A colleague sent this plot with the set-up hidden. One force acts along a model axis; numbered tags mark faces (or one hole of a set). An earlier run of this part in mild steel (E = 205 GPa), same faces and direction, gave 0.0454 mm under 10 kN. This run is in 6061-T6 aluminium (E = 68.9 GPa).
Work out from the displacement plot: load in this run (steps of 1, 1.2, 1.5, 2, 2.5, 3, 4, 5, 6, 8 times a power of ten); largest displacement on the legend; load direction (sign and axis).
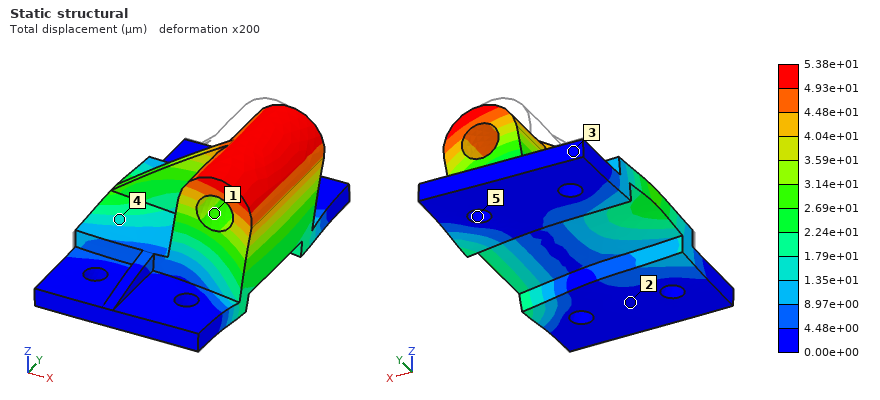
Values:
4 kN
5.38e+01 µm
+X
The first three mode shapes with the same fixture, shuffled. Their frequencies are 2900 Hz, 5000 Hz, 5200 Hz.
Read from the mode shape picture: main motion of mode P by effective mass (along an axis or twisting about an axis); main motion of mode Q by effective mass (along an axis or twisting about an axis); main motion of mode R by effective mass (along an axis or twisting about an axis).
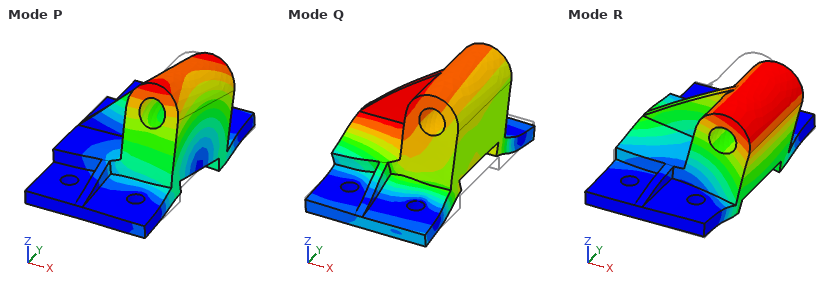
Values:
along Y
along Z
along X
